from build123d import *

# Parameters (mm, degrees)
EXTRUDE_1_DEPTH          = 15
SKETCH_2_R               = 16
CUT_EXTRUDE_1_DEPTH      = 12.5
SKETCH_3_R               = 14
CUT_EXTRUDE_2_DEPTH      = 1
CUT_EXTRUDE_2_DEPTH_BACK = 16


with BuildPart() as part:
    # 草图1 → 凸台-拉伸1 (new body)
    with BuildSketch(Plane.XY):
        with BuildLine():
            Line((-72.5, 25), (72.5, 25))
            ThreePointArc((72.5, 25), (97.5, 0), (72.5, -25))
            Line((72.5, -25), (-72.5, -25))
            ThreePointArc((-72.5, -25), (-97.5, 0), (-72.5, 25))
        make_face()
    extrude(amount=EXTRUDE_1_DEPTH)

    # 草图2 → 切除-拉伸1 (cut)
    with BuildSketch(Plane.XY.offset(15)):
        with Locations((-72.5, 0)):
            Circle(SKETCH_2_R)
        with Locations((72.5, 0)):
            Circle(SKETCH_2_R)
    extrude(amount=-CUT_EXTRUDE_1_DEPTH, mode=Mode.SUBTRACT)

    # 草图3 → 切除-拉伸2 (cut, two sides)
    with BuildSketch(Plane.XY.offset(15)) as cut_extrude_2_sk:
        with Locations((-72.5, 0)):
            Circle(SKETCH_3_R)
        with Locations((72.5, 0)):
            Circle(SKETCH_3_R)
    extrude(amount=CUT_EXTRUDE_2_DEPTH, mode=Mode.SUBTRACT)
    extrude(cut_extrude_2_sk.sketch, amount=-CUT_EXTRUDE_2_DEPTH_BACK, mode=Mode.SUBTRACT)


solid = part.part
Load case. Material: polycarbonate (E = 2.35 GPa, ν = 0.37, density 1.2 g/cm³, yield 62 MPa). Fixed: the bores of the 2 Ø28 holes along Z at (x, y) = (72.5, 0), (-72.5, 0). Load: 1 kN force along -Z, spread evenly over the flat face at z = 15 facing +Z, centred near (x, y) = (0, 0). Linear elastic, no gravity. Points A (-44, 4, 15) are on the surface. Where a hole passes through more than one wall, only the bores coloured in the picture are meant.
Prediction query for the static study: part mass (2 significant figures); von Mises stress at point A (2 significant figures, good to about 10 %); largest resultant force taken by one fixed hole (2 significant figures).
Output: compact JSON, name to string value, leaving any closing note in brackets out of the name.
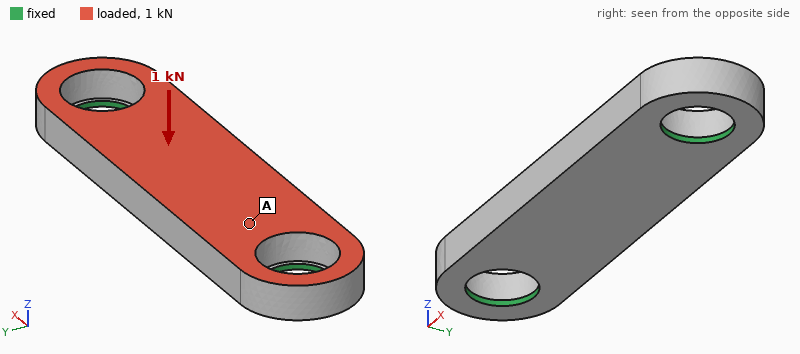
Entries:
{"part mass": "140 g", "von Mises stress at point A": "1.5 MPa", "largest resultant force taken by one fixed hole": "720 N"}
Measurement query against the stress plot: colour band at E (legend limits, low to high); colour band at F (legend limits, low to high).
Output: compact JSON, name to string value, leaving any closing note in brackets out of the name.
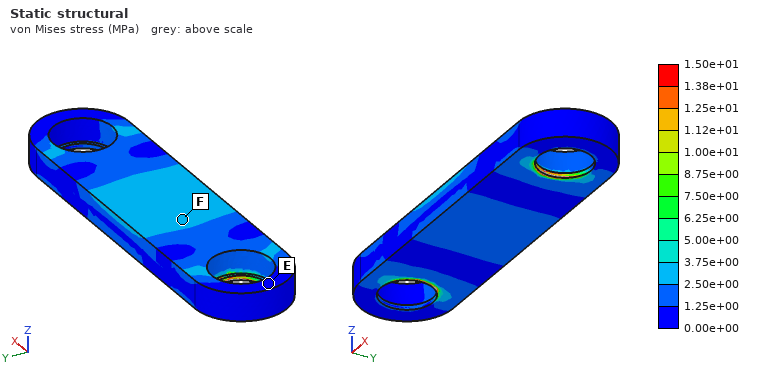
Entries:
{"colour band at E": "0.00e+00 to 1.25e+00 MPa", "colour band at F": "2.50e+00 to 3.75e+00 MPa"}
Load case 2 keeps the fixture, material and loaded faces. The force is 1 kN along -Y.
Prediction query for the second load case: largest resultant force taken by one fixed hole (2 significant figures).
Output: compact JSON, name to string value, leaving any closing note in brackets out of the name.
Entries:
{"largest resultant force taken by one fixed hole": "500 N"}
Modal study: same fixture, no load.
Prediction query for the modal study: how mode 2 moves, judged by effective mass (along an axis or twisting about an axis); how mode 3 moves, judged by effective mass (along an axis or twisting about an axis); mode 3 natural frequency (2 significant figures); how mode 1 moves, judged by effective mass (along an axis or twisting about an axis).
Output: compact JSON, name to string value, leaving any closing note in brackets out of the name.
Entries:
{"how mode 2 moves, judged by effective mass": "along Y", "how mode 3 moves, judged by effective mass": "along Y", "mode 3 natural frequency": "1800 Hz", "how mode 1 moves, judged by effective mass": "along Z"}
